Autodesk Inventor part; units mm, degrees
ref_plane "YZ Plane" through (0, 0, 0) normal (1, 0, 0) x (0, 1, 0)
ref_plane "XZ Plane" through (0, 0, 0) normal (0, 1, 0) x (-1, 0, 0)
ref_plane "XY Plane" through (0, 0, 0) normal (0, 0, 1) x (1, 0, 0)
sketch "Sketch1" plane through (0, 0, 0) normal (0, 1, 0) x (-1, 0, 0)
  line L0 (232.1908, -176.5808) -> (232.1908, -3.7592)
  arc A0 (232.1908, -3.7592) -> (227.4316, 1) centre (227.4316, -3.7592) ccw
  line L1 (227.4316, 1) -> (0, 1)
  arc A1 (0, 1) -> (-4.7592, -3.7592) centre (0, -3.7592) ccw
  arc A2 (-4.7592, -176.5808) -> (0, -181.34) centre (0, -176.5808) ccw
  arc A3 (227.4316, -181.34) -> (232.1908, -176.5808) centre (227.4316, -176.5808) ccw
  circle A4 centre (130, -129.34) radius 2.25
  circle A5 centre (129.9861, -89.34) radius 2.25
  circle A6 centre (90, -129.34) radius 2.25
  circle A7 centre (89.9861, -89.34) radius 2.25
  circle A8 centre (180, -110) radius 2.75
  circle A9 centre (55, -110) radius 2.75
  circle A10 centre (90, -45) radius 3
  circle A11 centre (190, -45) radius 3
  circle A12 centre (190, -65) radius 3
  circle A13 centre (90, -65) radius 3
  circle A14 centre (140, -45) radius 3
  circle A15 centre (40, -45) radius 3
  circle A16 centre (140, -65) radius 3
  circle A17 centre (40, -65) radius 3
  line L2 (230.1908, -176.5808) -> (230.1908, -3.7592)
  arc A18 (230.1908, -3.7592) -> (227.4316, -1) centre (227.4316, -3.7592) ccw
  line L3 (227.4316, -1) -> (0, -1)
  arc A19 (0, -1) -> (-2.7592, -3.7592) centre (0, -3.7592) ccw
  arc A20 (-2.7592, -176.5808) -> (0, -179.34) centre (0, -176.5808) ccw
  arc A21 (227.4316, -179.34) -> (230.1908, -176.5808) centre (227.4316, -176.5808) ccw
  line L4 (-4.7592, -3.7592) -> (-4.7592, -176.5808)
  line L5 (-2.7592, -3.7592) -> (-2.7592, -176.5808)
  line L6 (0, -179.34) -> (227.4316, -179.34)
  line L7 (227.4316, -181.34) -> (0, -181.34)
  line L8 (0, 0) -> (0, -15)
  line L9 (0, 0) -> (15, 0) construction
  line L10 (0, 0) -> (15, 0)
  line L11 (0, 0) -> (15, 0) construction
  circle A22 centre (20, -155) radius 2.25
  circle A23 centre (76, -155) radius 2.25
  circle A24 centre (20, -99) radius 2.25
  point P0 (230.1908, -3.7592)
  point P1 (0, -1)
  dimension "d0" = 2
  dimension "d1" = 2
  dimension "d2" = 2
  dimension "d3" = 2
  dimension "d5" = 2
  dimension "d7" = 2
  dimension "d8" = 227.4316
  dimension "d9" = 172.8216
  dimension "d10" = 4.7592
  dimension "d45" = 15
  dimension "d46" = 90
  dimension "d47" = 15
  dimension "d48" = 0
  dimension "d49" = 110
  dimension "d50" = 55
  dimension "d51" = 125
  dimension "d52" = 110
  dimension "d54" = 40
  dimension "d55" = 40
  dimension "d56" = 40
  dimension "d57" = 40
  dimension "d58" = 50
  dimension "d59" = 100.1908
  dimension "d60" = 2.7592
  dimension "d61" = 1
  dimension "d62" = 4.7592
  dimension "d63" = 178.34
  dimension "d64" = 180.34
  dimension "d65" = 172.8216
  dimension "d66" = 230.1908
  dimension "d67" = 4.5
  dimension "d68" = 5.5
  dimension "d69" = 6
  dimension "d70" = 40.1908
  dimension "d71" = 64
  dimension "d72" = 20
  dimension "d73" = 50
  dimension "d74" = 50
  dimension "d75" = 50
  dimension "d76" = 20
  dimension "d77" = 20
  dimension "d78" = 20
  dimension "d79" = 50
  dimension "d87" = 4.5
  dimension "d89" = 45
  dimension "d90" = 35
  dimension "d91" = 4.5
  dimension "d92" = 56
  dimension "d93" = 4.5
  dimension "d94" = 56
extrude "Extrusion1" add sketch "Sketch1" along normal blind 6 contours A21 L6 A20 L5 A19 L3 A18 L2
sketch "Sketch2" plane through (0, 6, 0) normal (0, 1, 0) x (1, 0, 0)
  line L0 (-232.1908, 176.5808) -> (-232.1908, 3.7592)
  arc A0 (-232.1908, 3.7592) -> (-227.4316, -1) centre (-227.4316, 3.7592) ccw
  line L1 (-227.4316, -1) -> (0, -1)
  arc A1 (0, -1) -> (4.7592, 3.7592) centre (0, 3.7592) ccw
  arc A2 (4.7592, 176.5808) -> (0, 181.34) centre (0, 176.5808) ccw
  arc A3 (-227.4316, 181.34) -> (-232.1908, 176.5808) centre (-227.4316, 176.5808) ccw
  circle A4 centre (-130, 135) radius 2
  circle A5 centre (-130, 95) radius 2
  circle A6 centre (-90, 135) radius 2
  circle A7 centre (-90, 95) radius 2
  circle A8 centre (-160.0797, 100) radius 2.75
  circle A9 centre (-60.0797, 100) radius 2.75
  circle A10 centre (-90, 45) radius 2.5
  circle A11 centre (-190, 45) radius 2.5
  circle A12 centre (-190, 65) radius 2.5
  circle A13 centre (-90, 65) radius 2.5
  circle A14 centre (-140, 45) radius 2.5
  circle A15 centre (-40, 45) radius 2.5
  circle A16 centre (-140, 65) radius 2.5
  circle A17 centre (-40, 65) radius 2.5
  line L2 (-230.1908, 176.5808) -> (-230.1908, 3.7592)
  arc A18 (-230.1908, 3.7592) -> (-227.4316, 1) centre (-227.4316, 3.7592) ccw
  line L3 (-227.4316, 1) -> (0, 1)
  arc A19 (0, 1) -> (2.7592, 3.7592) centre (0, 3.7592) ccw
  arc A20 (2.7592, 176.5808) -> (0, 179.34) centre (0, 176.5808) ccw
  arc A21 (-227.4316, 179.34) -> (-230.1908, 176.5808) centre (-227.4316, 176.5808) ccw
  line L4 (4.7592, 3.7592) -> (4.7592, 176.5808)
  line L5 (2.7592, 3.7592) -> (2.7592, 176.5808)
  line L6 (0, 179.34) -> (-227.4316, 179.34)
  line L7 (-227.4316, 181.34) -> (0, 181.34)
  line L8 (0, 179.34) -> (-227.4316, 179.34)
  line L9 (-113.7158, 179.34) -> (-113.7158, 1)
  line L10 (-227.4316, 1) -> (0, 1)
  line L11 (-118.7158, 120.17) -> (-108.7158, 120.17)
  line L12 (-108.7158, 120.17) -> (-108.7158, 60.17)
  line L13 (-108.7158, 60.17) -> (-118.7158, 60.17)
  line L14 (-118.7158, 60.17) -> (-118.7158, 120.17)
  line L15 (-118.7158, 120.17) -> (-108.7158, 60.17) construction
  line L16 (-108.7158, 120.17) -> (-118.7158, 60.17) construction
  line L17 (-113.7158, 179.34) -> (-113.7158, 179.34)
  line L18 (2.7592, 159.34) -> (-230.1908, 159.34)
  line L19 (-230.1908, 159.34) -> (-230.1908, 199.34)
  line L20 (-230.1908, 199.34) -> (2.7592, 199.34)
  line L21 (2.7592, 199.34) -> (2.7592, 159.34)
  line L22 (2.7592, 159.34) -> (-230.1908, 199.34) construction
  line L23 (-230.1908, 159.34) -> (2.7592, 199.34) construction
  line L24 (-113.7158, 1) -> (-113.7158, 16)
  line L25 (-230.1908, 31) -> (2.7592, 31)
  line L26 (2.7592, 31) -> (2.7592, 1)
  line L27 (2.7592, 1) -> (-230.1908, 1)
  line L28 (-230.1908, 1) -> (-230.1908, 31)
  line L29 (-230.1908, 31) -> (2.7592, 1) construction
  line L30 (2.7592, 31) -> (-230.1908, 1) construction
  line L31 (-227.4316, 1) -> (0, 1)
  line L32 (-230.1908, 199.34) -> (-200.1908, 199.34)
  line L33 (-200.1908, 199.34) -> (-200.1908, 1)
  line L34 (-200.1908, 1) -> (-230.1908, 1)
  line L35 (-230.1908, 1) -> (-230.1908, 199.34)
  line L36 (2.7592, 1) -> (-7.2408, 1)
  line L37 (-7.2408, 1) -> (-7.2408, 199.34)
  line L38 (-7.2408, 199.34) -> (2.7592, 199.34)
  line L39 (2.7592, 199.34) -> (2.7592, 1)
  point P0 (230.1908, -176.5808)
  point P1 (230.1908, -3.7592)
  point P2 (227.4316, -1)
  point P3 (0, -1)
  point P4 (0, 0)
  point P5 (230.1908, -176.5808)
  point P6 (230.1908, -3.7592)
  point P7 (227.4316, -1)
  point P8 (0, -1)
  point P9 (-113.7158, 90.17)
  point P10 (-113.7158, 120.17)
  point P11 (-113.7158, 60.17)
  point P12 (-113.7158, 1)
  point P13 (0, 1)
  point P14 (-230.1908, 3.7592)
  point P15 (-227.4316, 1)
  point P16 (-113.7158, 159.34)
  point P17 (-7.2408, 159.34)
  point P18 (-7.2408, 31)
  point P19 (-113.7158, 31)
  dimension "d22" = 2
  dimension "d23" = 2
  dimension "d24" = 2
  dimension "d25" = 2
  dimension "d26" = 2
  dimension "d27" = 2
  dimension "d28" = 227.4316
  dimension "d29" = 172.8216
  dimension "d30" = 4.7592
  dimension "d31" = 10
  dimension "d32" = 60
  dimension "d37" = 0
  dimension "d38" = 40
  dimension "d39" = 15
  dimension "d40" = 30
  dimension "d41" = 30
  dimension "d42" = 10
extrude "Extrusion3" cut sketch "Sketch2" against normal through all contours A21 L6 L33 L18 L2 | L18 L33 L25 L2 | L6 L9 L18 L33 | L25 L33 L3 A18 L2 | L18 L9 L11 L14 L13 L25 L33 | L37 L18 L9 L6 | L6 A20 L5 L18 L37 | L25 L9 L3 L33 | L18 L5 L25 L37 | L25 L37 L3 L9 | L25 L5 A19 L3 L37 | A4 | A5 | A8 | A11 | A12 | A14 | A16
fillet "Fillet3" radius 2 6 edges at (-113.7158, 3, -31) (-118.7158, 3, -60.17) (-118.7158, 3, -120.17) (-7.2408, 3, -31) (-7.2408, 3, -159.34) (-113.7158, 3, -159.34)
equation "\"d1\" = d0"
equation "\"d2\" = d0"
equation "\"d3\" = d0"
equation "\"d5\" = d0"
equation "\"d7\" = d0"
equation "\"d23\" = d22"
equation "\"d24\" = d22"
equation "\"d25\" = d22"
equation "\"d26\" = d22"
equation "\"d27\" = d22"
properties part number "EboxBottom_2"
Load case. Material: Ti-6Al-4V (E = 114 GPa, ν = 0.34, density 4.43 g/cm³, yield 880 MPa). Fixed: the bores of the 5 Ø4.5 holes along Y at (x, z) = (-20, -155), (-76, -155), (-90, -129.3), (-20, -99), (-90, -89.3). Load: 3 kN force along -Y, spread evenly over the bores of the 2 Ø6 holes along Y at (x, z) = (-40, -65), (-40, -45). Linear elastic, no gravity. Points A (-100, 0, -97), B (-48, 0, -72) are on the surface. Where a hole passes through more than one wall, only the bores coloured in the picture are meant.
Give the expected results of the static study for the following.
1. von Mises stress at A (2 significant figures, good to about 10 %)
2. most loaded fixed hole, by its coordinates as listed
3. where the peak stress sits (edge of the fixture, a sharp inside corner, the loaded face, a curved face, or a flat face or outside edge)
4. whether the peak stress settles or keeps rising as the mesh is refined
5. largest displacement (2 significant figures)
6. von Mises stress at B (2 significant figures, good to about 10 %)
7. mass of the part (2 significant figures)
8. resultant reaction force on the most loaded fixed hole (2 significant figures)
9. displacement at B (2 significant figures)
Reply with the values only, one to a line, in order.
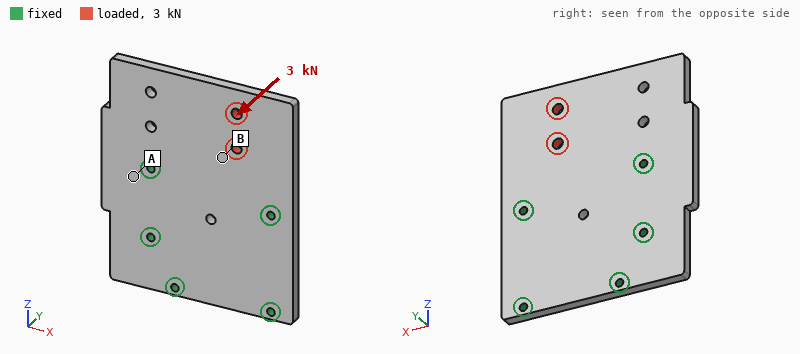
38 MPa
(-20, -99)
edge of the fixture
keeps rising
0.97 mm
110 MPa
370 g
2.4 kN
0.27 mm
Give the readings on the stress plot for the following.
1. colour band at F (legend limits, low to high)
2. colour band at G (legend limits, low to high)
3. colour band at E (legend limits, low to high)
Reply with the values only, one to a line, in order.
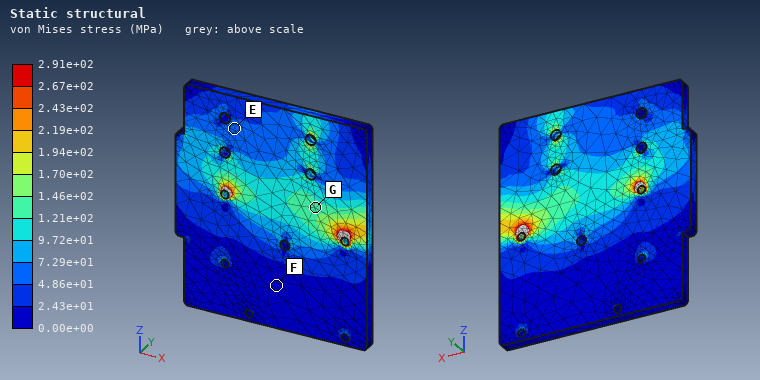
0.00e+00 to 2.43e+01 MPa
1.21e+02 to 1.46e+02 MPa
4.86e+01 to 7.29e+01 MPa
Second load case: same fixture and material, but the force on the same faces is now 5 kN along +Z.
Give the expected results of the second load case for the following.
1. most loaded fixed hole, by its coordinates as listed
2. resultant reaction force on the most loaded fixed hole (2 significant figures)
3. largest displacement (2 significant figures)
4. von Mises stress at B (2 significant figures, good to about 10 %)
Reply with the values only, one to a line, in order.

(-20, -99)
2.8 kN
9.9 µm
16 MPa
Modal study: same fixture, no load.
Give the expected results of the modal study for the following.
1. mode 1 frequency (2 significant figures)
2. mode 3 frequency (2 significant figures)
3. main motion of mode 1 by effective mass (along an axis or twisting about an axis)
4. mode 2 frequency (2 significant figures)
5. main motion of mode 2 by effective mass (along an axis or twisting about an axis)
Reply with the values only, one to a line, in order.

1100 Hz
3700 Hz
along Y
2000 Hz
twisting about Z
